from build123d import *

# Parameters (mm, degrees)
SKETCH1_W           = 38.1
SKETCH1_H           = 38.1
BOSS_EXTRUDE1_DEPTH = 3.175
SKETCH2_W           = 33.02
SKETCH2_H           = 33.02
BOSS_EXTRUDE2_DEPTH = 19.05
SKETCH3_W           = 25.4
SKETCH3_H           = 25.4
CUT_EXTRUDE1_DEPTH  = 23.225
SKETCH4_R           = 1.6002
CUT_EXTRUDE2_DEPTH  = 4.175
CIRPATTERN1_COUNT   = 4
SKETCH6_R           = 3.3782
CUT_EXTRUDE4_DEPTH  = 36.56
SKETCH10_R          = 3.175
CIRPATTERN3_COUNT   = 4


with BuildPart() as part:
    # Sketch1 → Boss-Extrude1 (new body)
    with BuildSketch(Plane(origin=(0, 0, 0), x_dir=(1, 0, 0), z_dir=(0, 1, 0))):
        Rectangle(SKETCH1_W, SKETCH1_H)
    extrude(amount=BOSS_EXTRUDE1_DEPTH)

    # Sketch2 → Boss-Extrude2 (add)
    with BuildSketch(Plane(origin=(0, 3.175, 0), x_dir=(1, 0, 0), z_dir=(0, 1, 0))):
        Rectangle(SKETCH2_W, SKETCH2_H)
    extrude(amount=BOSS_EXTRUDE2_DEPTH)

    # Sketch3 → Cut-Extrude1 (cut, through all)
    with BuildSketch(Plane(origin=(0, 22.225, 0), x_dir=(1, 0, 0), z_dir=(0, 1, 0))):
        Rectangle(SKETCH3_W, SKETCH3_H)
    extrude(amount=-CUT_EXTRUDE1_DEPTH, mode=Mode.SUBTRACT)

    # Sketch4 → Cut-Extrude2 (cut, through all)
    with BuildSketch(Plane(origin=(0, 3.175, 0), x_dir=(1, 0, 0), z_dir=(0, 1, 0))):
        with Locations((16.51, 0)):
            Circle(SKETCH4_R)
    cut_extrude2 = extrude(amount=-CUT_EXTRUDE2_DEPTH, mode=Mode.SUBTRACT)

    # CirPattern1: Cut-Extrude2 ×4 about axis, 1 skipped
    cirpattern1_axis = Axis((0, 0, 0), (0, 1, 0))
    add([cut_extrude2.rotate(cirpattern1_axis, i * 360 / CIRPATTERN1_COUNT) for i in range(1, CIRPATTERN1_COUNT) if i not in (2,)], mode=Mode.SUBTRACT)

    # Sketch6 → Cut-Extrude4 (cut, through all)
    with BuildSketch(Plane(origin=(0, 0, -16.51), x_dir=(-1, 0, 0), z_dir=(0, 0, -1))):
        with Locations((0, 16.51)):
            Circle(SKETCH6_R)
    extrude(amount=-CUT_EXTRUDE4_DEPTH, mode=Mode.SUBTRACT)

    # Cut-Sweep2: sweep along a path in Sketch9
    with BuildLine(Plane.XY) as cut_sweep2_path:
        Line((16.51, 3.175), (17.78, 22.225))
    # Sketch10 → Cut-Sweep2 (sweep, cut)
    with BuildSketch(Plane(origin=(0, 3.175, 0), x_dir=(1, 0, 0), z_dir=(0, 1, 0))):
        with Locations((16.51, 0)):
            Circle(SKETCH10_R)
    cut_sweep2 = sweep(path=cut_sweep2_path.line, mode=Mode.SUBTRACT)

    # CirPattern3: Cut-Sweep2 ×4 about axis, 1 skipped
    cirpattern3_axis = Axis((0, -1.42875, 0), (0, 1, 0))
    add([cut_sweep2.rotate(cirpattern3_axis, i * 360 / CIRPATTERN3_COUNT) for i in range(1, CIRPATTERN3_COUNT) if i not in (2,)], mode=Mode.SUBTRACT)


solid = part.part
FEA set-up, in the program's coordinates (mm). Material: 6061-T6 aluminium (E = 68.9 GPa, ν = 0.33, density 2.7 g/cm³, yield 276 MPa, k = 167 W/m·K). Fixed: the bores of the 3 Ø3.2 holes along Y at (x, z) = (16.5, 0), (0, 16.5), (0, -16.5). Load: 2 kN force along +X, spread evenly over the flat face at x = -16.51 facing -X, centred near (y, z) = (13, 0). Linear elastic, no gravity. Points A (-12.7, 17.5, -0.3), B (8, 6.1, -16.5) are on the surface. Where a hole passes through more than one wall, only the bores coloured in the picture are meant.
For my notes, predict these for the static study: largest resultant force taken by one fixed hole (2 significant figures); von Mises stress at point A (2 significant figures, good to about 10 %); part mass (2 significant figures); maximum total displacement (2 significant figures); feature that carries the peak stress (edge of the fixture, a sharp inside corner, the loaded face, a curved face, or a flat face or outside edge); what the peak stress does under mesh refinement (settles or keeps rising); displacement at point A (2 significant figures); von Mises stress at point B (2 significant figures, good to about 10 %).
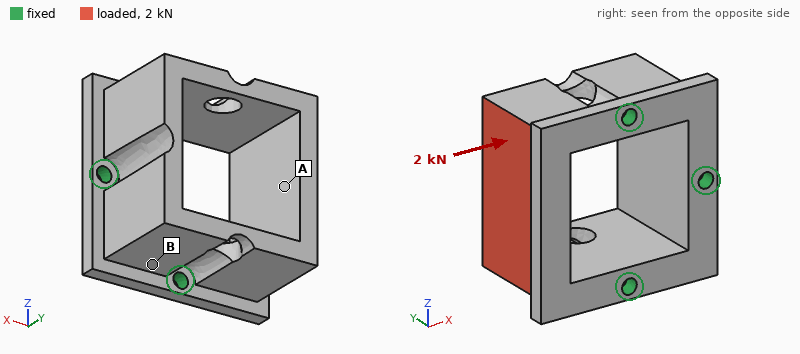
1.2 kN
55 MPa
27 g
96 µm
edge of the fixture
keeps rising
75 µm
21 MPa
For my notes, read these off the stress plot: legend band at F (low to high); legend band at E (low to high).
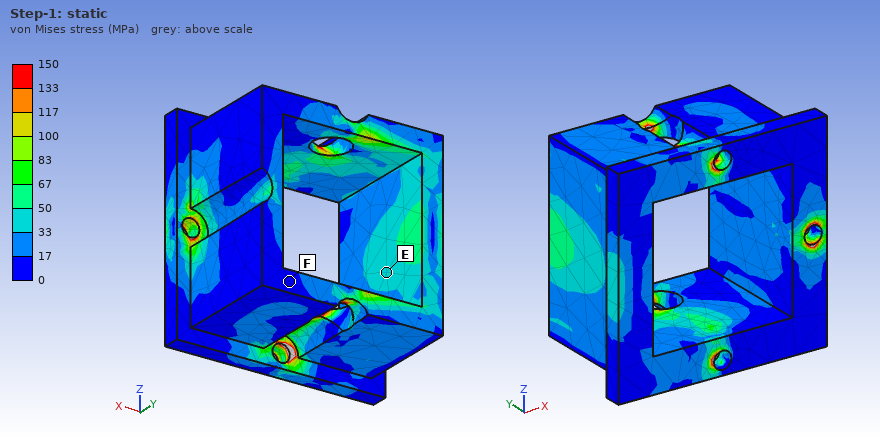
0 to 17 MPa
33 to 50 MPa
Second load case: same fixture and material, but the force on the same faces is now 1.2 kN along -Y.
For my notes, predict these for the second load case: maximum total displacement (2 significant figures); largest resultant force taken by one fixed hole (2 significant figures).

66 µm
1.1 kN
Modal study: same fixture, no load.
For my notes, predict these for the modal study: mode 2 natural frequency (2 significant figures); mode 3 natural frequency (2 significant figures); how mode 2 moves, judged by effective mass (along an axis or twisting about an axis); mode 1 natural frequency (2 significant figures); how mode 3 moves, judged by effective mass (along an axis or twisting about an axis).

7500 Hz
8500 Hz
along Z
6700 Hz
along Z
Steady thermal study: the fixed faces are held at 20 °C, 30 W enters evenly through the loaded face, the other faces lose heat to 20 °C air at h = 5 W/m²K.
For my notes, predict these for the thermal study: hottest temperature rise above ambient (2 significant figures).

33 K
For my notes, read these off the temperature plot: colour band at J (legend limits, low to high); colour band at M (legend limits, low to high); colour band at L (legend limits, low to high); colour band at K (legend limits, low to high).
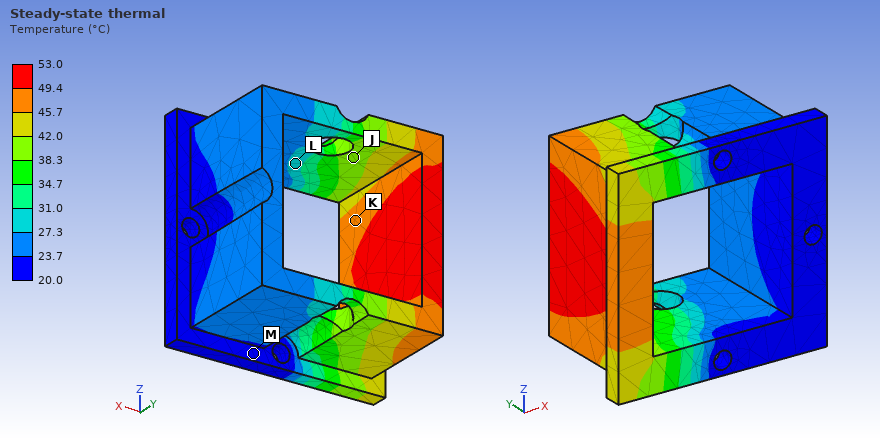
38.3 to 42.0 °C
20.0 to 23.7 °C
27.3 to 31.0 °C
45.7 to 49.4 °C
